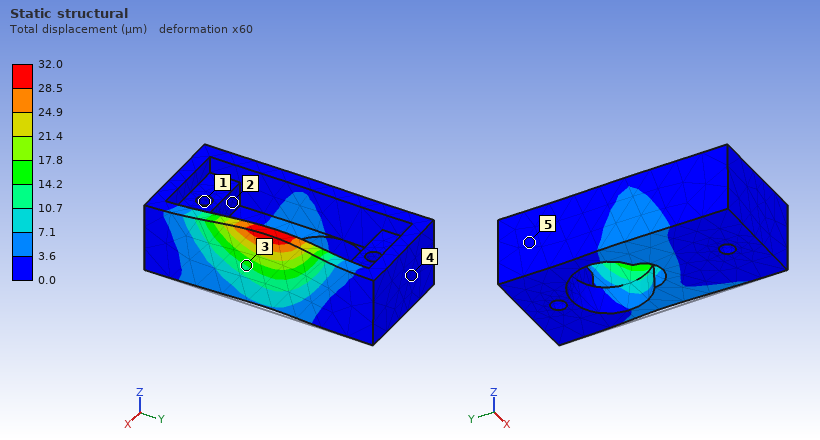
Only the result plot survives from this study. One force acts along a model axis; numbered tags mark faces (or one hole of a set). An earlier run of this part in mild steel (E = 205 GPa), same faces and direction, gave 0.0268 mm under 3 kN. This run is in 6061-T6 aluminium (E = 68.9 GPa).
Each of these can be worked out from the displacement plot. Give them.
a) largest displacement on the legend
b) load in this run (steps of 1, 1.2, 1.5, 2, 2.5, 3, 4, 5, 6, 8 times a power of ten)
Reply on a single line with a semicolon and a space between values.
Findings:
32.0 µm; 1.2 kN
